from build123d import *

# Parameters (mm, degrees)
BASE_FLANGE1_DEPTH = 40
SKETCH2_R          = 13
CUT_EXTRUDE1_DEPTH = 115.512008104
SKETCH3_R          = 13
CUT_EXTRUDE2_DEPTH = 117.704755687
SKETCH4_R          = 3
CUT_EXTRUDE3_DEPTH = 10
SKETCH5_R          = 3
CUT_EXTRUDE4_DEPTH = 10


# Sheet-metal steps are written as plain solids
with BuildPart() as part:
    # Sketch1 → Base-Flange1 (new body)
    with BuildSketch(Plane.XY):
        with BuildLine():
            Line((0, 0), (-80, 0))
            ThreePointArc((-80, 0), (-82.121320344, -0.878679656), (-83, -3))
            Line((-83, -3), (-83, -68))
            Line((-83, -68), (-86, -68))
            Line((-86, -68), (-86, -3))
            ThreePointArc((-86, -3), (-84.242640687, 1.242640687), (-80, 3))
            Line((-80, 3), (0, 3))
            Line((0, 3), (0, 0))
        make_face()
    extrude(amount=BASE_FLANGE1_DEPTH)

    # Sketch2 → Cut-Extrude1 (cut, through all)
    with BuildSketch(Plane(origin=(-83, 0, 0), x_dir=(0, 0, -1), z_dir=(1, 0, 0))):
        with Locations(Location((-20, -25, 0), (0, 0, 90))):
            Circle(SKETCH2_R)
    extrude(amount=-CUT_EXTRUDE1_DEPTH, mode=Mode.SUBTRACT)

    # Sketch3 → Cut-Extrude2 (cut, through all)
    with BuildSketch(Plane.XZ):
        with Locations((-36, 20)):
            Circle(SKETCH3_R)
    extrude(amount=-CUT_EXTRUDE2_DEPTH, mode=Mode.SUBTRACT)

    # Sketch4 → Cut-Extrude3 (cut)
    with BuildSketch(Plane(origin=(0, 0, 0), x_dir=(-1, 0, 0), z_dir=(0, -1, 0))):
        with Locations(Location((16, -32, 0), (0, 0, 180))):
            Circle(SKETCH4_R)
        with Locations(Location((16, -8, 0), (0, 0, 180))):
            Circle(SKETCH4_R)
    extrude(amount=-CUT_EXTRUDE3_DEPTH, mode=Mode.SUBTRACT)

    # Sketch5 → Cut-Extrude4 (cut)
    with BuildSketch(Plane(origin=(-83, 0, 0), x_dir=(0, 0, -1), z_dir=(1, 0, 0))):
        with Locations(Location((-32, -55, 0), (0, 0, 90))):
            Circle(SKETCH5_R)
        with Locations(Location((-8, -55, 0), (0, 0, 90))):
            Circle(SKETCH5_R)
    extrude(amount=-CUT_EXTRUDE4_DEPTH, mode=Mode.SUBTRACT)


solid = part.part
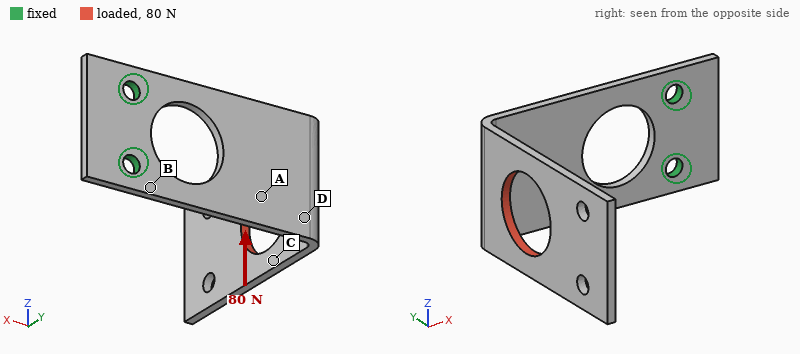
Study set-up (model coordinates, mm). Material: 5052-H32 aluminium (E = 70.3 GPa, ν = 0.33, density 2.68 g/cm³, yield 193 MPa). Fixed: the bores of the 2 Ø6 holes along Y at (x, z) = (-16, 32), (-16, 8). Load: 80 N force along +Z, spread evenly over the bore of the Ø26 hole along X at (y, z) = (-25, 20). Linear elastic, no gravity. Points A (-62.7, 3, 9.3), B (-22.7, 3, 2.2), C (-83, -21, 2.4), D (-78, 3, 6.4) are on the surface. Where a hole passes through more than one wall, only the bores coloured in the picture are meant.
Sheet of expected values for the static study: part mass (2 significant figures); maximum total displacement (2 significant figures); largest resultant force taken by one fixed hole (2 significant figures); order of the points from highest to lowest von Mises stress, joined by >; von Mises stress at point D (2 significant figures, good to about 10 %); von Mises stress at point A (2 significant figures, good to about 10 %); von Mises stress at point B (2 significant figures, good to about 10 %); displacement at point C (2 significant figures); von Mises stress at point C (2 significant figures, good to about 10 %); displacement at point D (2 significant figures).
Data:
39 g
1.2 mm
190 N
B > A > D > C
25 MPa
33 MPa
50 MPa
0.49 mm
7.3 MPa
0.21 mm
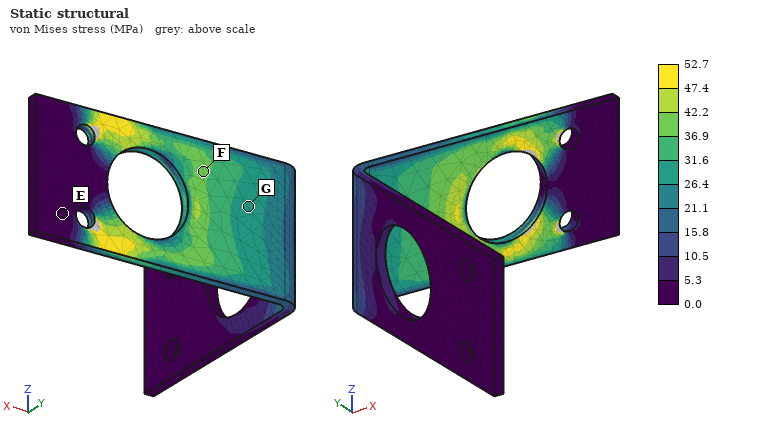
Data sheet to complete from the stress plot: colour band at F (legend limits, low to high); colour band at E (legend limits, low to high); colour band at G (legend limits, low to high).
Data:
36.9 to 42.2 MPa
0.0 to 5.3 MPa
26.4 to 31.6 MPa
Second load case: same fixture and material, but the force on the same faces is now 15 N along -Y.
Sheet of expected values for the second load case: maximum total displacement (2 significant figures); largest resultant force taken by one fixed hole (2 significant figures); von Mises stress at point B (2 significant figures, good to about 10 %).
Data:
0.82 mm
7.5 N
23 MPa
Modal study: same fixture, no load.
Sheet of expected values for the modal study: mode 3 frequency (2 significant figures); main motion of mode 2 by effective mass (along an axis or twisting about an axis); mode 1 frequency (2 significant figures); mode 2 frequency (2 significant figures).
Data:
450 Hz
along Z
150 Hz
300 Hz
